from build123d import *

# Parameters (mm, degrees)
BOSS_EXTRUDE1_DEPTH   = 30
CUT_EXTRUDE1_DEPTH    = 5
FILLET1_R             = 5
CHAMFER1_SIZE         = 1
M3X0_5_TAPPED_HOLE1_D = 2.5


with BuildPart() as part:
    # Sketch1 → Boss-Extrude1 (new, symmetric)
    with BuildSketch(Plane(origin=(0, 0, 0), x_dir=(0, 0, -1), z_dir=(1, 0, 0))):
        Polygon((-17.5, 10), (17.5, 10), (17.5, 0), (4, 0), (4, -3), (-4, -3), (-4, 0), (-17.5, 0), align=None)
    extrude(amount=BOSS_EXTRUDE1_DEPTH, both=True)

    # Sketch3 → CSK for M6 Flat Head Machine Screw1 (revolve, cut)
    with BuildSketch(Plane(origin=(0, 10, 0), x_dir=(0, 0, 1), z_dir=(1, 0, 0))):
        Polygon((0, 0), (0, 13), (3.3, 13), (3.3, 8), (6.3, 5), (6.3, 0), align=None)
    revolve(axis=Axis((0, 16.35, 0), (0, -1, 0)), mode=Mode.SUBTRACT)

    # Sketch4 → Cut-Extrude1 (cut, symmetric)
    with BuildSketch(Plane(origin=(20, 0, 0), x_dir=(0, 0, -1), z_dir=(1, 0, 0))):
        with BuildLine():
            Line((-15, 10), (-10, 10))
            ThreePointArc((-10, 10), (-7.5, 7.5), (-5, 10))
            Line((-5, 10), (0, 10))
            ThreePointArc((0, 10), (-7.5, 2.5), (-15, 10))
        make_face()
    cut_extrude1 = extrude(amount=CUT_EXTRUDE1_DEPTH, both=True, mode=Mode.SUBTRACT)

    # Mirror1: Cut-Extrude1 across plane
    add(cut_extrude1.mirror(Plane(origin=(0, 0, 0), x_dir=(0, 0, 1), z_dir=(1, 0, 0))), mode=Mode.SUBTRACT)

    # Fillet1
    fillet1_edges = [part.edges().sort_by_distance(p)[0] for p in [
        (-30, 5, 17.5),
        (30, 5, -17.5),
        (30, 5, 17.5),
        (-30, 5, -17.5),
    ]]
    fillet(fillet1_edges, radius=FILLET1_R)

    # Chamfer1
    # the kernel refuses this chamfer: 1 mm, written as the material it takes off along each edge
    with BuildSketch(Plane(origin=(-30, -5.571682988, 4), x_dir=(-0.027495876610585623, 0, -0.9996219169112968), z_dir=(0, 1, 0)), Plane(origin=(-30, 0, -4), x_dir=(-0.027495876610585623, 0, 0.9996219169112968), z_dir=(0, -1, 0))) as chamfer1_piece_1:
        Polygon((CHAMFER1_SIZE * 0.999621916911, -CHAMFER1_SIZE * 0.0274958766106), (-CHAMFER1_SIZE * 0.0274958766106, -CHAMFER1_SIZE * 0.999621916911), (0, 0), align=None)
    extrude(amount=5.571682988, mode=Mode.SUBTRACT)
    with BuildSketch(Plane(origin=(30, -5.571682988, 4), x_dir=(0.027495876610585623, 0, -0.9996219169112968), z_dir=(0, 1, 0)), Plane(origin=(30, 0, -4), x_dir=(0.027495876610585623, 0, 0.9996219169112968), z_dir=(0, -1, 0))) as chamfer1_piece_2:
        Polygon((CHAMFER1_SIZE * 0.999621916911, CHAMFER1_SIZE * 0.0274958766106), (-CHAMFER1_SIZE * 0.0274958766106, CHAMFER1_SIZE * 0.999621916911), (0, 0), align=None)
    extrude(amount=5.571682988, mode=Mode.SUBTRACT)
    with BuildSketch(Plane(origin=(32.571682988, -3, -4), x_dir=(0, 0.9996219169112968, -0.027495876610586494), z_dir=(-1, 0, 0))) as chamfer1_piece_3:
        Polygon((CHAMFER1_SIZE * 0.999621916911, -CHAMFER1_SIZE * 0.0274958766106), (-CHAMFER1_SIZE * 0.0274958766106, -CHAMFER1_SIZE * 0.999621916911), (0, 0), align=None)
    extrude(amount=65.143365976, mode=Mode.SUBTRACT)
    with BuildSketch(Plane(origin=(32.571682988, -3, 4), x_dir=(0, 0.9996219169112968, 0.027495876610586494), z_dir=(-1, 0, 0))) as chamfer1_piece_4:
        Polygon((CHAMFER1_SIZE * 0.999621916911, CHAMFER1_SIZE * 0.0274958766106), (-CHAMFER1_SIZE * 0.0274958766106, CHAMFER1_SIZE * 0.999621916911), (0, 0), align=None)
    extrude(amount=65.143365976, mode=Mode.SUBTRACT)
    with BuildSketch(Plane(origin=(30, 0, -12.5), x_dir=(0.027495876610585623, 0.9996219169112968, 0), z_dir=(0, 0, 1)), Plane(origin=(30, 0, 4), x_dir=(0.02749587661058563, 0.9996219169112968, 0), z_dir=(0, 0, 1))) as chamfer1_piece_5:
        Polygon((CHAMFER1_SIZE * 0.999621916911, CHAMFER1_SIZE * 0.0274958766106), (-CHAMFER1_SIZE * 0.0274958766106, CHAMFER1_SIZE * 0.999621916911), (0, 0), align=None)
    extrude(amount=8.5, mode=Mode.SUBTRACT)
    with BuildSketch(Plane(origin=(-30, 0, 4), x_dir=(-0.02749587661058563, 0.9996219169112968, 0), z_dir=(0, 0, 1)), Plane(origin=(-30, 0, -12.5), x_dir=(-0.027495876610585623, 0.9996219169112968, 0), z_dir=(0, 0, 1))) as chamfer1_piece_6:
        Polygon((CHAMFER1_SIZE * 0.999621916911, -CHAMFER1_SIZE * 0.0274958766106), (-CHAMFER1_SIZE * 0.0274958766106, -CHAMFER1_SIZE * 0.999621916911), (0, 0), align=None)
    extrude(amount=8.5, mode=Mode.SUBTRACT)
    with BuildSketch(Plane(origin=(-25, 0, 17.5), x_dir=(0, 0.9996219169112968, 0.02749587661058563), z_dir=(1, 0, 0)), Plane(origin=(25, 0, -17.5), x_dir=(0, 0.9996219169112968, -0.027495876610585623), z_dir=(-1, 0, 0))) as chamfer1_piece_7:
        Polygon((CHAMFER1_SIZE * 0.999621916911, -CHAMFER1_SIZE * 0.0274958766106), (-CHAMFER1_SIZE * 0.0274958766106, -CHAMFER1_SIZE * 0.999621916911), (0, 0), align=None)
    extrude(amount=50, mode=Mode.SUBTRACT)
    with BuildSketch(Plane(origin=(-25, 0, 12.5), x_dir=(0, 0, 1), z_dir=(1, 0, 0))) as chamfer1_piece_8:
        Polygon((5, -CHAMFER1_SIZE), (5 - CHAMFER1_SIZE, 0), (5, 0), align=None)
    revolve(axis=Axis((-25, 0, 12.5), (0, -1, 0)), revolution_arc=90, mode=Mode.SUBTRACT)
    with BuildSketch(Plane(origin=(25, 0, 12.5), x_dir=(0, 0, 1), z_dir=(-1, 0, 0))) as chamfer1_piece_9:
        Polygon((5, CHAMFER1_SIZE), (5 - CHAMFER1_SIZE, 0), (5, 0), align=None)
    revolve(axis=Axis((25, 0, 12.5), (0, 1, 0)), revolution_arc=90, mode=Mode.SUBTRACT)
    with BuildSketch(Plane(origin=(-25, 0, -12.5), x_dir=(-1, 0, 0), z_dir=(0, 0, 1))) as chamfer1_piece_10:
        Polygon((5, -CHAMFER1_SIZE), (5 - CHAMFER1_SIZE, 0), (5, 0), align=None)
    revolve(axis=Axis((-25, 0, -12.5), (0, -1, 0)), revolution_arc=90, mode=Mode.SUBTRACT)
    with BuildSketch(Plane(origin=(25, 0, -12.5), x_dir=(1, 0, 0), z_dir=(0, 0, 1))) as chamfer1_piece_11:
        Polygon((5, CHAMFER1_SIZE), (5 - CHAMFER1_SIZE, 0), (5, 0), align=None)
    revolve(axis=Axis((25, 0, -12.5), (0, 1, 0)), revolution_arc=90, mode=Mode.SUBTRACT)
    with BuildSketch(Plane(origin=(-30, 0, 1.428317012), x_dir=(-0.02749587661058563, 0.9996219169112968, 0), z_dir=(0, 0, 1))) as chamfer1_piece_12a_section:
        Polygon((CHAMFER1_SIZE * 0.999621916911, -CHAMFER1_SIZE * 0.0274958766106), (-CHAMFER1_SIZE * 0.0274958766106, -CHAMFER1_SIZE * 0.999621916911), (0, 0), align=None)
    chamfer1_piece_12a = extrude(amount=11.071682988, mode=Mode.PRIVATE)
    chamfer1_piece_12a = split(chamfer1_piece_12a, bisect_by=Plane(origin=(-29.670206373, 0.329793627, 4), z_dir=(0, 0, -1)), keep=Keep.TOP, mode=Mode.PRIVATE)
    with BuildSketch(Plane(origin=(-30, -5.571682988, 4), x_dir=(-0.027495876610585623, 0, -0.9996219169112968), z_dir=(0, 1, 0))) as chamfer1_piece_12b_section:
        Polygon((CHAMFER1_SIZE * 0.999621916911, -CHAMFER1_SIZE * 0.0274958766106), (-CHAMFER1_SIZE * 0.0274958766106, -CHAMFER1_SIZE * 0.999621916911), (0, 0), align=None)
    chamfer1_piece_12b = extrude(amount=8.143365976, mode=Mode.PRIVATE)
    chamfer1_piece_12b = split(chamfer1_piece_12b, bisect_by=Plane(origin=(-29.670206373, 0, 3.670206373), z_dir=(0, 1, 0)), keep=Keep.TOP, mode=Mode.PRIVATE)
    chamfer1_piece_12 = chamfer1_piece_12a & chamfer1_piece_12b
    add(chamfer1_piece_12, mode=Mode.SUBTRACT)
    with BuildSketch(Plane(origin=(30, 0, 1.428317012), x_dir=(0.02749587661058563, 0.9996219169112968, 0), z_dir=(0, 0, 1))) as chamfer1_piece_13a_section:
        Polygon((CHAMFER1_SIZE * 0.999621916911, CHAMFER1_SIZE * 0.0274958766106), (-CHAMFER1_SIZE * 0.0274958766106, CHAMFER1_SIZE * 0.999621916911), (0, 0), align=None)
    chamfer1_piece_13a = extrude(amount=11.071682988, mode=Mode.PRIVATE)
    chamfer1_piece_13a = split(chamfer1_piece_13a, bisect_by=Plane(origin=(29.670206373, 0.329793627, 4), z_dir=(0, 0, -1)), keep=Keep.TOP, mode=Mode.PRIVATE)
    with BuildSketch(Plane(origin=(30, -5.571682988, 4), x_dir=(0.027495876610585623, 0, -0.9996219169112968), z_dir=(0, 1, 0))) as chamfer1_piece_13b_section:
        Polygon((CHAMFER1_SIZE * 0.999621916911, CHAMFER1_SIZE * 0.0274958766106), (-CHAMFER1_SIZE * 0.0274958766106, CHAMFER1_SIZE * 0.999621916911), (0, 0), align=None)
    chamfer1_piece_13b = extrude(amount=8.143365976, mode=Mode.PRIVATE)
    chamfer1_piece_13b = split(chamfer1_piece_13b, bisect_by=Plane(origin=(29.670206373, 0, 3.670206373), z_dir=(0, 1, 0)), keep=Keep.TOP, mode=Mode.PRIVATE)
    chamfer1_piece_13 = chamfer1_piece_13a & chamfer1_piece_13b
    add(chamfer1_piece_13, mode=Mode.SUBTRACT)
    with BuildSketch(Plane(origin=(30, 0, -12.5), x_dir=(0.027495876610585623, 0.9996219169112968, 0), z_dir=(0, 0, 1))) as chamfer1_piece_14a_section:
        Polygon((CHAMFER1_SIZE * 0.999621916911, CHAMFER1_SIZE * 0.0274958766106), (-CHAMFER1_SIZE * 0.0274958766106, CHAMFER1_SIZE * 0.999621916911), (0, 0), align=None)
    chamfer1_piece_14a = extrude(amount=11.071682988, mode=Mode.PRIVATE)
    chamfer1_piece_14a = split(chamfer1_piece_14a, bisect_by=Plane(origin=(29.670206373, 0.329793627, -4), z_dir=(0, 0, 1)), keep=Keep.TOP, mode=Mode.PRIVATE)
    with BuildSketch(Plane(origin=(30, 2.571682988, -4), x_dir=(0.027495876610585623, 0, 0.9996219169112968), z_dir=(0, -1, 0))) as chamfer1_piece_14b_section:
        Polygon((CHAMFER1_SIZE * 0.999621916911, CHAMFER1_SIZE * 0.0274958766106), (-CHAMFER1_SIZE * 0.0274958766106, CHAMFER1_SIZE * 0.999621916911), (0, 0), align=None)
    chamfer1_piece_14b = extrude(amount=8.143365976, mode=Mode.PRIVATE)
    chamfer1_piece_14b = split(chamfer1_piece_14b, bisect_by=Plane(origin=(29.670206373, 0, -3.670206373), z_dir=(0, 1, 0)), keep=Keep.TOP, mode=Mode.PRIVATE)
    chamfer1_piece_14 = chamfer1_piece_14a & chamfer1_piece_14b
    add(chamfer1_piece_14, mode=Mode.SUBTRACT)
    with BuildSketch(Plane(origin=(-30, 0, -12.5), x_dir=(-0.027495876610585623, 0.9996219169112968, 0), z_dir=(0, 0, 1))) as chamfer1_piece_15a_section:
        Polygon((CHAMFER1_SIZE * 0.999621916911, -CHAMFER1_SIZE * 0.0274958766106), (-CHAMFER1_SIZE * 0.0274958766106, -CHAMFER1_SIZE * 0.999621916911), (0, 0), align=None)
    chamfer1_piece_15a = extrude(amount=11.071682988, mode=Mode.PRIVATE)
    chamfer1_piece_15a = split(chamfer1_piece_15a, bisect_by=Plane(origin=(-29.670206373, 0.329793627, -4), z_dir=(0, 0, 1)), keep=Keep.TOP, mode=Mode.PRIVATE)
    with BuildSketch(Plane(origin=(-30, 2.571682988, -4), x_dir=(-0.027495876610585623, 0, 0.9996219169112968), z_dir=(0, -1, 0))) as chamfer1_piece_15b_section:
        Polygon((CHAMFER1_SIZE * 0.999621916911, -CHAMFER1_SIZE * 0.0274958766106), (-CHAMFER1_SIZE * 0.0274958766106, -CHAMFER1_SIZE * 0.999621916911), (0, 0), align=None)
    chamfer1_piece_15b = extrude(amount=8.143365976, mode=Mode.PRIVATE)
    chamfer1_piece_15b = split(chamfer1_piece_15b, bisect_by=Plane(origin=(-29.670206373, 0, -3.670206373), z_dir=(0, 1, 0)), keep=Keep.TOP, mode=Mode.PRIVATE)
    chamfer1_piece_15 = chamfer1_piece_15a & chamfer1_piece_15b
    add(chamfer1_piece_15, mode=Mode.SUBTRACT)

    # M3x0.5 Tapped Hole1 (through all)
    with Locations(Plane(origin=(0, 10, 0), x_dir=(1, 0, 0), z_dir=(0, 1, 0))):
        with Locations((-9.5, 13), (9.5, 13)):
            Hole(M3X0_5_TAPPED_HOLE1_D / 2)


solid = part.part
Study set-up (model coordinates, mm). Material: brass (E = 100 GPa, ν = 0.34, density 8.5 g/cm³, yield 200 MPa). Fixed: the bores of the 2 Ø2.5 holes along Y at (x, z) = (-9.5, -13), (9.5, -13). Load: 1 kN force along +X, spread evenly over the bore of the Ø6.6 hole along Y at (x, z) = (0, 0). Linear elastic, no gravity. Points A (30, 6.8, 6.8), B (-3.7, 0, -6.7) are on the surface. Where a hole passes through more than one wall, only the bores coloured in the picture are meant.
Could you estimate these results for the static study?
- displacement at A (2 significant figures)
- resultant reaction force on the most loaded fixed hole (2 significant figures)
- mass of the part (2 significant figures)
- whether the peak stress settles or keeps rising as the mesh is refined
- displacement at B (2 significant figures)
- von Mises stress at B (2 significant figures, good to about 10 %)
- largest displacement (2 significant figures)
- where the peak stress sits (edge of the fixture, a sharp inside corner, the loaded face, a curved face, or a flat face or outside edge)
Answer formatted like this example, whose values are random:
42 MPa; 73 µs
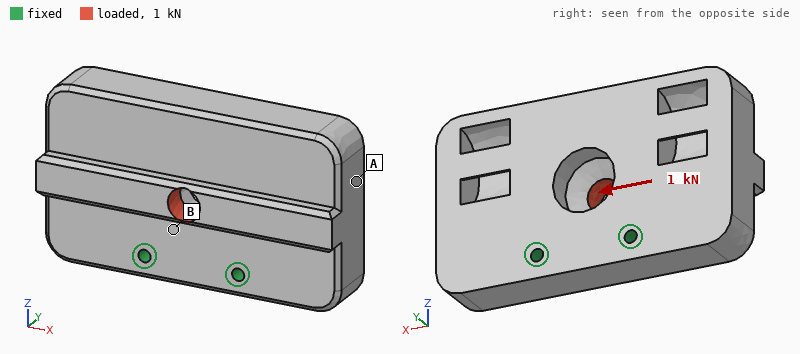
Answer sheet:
5.0 µm; 810 N; 160 g; keeps rising; 1.3 µm; 14 MPa; 6.0 µm; a sharp inside corner
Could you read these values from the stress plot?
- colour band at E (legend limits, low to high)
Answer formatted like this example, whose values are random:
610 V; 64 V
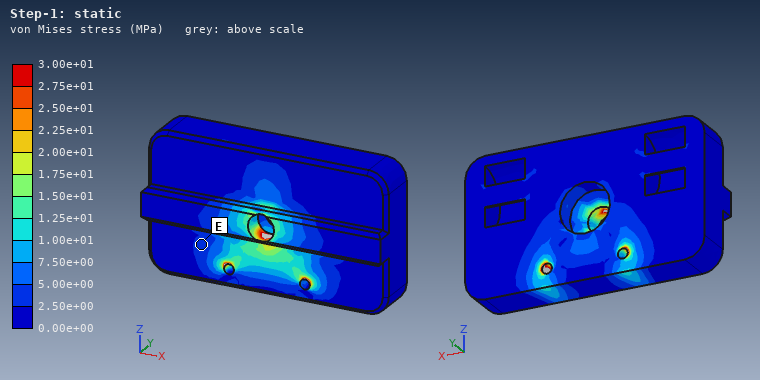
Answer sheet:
2.50e+00 to 5.00e+00 MPa
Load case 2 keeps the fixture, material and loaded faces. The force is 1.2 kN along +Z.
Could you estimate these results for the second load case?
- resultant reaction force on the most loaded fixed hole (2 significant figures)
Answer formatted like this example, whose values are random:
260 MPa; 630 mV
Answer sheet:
620 N
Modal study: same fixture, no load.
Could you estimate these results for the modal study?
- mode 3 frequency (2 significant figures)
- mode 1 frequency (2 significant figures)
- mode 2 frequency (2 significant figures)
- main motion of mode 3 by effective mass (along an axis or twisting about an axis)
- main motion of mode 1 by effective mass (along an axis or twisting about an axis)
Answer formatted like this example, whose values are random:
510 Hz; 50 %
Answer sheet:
5800 Hz; 3900 Hz; 5000 Hz; along X; along Y
